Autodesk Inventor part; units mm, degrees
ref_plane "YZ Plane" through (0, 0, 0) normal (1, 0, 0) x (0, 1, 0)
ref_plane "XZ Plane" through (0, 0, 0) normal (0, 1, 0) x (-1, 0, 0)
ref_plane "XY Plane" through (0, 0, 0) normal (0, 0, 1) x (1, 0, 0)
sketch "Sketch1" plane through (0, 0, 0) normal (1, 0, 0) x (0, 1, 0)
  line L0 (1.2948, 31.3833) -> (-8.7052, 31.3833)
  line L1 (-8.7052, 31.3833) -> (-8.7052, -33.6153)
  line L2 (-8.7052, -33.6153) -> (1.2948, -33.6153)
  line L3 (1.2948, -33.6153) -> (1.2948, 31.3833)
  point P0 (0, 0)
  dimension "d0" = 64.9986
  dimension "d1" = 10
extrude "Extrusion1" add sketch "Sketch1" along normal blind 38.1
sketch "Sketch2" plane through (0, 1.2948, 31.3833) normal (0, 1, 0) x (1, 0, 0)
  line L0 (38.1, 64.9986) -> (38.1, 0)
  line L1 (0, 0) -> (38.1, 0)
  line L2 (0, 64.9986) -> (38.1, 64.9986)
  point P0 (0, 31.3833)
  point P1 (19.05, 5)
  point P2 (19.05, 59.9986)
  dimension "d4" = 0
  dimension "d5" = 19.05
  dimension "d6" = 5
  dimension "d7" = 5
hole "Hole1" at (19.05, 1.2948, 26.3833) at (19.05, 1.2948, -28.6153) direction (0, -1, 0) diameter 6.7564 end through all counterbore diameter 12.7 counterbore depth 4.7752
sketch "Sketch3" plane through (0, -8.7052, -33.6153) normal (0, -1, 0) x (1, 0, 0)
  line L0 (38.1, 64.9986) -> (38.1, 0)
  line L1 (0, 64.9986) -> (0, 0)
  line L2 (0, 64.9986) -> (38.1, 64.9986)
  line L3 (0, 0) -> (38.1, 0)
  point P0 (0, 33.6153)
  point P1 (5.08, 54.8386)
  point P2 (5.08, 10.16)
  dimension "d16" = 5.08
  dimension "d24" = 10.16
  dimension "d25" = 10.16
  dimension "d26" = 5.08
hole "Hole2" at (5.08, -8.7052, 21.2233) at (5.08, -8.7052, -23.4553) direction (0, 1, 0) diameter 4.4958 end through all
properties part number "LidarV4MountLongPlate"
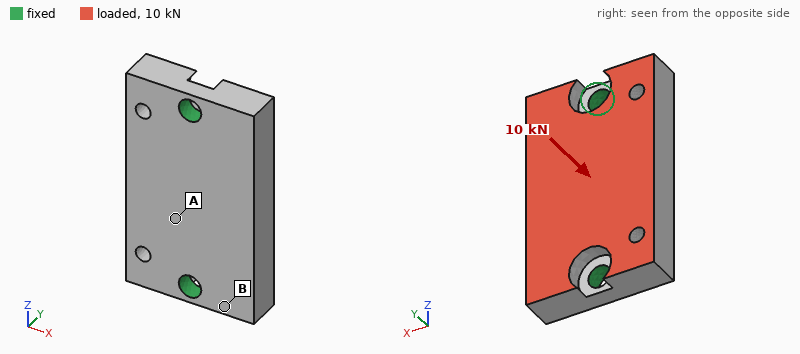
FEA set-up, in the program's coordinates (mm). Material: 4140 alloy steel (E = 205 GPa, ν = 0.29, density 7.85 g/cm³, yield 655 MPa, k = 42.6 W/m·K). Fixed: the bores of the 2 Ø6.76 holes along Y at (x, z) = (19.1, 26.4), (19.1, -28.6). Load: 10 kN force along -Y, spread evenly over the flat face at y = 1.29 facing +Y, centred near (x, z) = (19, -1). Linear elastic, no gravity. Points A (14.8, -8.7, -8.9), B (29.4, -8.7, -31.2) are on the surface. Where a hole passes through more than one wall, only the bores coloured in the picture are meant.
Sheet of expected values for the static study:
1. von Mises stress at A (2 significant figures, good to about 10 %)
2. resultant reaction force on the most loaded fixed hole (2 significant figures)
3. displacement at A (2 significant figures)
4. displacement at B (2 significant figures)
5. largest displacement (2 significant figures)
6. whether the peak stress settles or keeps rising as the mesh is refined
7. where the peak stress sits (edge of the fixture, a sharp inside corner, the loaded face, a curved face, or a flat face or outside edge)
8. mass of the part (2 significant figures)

45 MPa
5.8 kN
16 µm
4.7 µm
23 µm
keeps rising
edge of the fixture
180 g
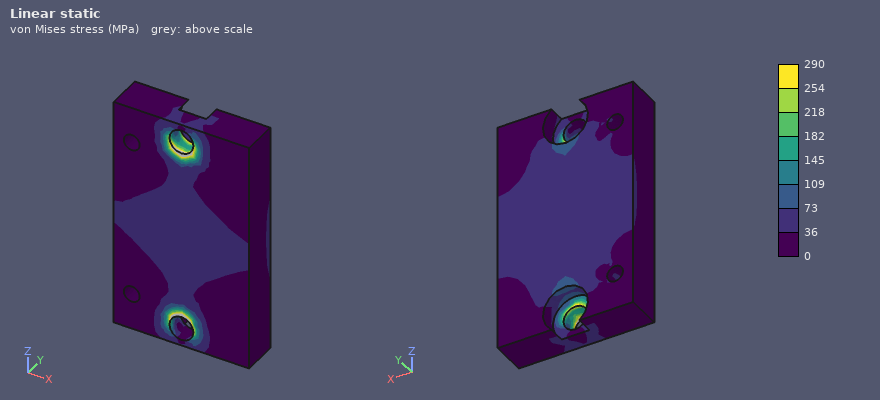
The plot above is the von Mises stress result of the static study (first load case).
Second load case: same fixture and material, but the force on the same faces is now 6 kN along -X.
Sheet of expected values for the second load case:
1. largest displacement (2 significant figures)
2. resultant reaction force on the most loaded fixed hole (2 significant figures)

26 µm
3.0 kN
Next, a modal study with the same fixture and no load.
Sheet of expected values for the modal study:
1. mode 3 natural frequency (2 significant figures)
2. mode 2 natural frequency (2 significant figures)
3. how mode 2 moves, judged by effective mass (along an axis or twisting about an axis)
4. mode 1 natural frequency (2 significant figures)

16 kHz
9500 Hz
along Y
6600 Hz
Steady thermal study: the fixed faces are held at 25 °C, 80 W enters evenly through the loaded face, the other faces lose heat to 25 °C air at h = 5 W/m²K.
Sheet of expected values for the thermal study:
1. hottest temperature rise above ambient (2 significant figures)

64 K
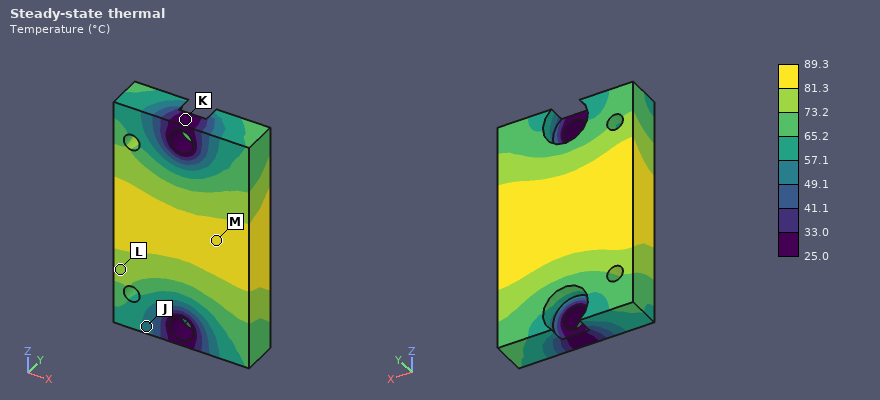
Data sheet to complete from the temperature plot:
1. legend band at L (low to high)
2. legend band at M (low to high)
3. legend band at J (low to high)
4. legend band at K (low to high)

73.2 to 81.3 °C
81.3 to 89.3 °C
49.1 to 57.1 °C
25.0 to 33.0 °C
